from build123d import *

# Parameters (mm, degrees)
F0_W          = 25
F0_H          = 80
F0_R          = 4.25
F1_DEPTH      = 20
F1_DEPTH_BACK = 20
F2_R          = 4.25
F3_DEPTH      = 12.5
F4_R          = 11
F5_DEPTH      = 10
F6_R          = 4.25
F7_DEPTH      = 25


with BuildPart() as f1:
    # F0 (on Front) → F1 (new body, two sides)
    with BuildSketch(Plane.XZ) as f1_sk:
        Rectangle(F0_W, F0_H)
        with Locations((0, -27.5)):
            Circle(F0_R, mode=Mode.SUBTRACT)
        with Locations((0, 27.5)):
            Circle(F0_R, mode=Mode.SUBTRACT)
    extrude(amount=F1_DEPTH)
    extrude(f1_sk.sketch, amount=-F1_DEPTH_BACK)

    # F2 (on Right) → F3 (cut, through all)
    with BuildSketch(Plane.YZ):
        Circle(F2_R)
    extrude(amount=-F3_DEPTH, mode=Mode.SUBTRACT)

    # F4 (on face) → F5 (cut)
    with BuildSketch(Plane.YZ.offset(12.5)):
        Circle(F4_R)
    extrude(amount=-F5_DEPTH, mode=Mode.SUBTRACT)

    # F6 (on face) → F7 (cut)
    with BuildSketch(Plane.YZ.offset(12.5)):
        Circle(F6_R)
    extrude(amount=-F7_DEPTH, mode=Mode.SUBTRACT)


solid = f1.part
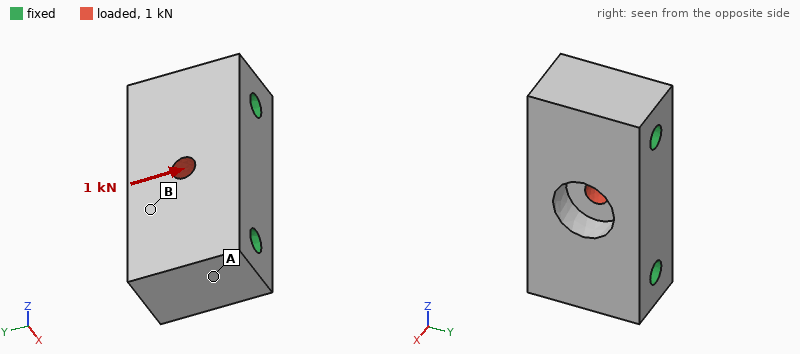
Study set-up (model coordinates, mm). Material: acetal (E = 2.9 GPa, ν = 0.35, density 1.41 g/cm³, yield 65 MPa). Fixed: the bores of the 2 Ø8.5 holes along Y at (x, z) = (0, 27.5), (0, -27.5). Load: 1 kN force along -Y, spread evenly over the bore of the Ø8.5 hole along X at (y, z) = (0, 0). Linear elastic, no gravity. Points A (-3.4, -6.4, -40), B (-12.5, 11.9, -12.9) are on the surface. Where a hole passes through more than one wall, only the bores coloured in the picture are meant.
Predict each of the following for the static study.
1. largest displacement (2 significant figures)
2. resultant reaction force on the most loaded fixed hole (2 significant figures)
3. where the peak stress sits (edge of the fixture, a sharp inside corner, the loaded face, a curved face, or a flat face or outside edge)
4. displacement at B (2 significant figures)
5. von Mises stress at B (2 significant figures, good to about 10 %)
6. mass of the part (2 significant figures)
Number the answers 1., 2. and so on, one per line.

1. 24 µm
2. 500 N
3. the loaded face
4. 12 µm
5. 1.6 MPa
6. 100 g
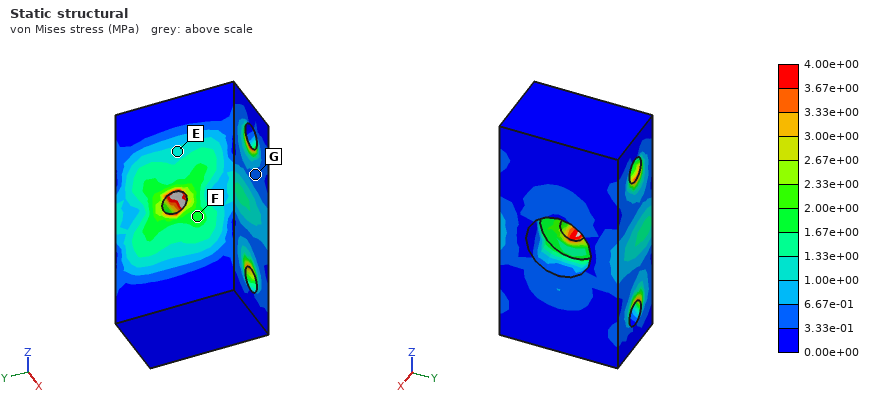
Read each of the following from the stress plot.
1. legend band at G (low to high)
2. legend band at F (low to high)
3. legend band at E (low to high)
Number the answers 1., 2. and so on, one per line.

1. 3.33e-01 to 6.67e-01 MPa
2. 1.67e+00 to 2.00e+00 MPa
3. 1.00e+00 to 1.33e+00 MPa
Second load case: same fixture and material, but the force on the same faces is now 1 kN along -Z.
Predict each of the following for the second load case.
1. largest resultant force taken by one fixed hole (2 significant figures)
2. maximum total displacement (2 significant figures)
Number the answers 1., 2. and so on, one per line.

1. 510 N
2. 12 µm
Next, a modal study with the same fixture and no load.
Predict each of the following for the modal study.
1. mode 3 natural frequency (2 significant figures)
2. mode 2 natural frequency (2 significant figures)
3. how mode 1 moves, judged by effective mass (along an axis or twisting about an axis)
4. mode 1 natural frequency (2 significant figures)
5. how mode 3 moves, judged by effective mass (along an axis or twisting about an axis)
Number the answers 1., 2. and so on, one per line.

1. 7800 Hz
2. 7300 Hz
3. along X
4. 5900 Hz
5. along Y
